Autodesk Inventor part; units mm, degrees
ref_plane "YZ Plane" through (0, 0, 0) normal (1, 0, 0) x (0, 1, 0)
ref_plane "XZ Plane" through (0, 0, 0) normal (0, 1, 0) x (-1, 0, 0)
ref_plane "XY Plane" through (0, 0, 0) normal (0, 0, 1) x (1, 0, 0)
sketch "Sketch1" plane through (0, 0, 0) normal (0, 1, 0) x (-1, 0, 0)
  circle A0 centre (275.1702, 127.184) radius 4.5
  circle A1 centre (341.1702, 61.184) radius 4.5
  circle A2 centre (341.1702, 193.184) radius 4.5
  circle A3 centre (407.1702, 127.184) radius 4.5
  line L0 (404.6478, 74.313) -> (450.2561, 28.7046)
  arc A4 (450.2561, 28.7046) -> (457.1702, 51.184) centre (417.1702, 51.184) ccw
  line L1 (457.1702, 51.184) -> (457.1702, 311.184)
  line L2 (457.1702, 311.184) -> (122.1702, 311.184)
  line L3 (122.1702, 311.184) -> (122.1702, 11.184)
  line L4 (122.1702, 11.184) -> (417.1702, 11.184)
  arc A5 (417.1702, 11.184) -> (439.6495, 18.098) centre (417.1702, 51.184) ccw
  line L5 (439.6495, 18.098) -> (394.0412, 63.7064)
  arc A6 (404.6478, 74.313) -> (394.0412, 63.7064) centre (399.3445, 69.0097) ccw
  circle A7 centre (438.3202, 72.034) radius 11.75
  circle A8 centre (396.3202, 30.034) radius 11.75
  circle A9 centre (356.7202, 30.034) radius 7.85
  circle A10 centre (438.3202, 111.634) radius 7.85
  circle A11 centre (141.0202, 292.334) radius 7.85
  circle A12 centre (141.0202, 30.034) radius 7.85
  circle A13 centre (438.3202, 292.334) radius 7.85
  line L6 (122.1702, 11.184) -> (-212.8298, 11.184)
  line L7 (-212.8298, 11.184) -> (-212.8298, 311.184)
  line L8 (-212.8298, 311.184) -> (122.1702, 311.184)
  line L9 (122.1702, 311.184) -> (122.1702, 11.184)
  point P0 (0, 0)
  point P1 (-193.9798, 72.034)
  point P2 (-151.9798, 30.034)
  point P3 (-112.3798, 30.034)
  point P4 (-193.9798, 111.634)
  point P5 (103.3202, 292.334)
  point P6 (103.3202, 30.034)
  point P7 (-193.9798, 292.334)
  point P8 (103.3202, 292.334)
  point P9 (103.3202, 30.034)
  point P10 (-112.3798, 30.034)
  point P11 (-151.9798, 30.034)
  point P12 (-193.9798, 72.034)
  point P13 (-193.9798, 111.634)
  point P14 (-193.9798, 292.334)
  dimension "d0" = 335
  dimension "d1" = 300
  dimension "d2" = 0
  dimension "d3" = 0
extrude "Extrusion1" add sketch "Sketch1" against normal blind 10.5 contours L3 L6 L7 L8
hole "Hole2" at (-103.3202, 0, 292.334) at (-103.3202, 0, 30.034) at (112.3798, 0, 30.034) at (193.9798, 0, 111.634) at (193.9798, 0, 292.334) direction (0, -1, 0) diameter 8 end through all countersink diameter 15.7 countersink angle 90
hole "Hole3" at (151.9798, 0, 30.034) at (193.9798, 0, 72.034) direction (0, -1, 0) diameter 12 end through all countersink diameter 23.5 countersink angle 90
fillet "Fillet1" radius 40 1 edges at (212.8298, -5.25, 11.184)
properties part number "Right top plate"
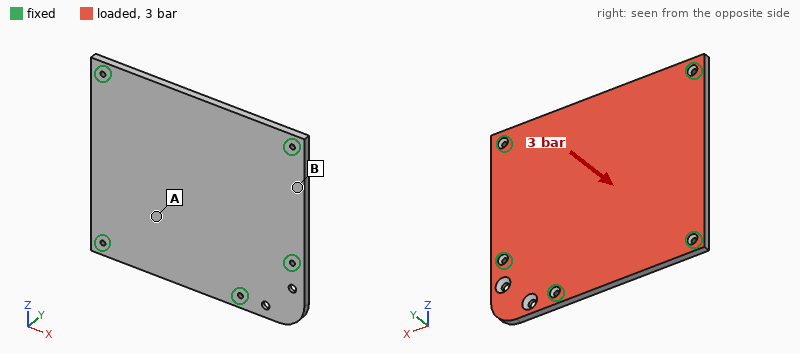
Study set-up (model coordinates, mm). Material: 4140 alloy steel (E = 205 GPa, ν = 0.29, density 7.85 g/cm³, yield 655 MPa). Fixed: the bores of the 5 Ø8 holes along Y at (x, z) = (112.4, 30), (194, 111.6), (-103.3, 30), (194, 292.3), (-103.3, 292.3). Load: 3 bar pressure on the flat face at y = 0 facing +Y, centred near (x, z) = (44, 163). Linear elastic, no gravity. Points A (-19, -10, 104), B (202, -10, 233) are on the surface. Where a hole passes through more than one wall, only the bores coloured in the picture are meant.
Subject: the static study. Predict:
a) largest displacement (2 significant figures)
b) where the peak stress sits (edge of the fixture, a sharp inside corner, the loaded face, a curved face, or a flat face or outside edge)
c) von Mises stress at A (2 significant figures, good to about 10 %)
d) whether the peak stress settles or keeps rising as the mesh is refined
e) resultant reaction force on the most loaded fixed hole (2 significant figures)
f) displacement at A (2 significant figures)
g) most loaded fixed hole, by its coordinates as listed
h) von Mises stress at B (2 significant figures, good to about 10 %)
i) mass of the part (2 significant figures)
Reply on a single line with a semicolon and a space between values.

0.63 mm; edge of the fixture; 49 MPa; keeps rising; 10 kN; 0.45 mm; (-103.3, 292.3); 30 MPa; 8.2 kg
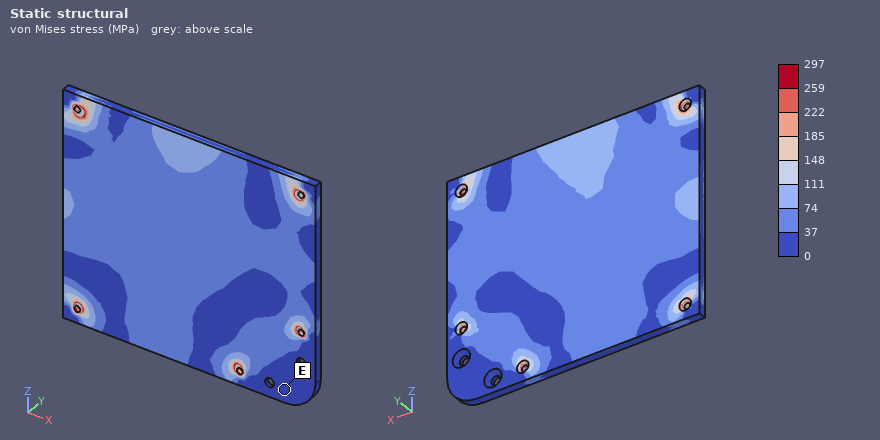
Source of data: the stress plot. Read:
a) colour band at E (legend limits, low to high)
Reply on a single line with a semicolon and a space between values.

0 to 37 MPa
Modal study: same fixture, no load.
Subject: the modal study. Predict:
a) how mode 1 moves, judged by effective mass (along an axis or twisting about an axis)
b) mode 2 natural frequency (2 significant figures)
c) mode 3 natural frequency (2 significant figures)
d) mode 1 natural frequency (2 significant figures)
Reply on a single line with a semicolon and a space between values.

along Y; 720 Hz; 970 Hz; 450 Hz
